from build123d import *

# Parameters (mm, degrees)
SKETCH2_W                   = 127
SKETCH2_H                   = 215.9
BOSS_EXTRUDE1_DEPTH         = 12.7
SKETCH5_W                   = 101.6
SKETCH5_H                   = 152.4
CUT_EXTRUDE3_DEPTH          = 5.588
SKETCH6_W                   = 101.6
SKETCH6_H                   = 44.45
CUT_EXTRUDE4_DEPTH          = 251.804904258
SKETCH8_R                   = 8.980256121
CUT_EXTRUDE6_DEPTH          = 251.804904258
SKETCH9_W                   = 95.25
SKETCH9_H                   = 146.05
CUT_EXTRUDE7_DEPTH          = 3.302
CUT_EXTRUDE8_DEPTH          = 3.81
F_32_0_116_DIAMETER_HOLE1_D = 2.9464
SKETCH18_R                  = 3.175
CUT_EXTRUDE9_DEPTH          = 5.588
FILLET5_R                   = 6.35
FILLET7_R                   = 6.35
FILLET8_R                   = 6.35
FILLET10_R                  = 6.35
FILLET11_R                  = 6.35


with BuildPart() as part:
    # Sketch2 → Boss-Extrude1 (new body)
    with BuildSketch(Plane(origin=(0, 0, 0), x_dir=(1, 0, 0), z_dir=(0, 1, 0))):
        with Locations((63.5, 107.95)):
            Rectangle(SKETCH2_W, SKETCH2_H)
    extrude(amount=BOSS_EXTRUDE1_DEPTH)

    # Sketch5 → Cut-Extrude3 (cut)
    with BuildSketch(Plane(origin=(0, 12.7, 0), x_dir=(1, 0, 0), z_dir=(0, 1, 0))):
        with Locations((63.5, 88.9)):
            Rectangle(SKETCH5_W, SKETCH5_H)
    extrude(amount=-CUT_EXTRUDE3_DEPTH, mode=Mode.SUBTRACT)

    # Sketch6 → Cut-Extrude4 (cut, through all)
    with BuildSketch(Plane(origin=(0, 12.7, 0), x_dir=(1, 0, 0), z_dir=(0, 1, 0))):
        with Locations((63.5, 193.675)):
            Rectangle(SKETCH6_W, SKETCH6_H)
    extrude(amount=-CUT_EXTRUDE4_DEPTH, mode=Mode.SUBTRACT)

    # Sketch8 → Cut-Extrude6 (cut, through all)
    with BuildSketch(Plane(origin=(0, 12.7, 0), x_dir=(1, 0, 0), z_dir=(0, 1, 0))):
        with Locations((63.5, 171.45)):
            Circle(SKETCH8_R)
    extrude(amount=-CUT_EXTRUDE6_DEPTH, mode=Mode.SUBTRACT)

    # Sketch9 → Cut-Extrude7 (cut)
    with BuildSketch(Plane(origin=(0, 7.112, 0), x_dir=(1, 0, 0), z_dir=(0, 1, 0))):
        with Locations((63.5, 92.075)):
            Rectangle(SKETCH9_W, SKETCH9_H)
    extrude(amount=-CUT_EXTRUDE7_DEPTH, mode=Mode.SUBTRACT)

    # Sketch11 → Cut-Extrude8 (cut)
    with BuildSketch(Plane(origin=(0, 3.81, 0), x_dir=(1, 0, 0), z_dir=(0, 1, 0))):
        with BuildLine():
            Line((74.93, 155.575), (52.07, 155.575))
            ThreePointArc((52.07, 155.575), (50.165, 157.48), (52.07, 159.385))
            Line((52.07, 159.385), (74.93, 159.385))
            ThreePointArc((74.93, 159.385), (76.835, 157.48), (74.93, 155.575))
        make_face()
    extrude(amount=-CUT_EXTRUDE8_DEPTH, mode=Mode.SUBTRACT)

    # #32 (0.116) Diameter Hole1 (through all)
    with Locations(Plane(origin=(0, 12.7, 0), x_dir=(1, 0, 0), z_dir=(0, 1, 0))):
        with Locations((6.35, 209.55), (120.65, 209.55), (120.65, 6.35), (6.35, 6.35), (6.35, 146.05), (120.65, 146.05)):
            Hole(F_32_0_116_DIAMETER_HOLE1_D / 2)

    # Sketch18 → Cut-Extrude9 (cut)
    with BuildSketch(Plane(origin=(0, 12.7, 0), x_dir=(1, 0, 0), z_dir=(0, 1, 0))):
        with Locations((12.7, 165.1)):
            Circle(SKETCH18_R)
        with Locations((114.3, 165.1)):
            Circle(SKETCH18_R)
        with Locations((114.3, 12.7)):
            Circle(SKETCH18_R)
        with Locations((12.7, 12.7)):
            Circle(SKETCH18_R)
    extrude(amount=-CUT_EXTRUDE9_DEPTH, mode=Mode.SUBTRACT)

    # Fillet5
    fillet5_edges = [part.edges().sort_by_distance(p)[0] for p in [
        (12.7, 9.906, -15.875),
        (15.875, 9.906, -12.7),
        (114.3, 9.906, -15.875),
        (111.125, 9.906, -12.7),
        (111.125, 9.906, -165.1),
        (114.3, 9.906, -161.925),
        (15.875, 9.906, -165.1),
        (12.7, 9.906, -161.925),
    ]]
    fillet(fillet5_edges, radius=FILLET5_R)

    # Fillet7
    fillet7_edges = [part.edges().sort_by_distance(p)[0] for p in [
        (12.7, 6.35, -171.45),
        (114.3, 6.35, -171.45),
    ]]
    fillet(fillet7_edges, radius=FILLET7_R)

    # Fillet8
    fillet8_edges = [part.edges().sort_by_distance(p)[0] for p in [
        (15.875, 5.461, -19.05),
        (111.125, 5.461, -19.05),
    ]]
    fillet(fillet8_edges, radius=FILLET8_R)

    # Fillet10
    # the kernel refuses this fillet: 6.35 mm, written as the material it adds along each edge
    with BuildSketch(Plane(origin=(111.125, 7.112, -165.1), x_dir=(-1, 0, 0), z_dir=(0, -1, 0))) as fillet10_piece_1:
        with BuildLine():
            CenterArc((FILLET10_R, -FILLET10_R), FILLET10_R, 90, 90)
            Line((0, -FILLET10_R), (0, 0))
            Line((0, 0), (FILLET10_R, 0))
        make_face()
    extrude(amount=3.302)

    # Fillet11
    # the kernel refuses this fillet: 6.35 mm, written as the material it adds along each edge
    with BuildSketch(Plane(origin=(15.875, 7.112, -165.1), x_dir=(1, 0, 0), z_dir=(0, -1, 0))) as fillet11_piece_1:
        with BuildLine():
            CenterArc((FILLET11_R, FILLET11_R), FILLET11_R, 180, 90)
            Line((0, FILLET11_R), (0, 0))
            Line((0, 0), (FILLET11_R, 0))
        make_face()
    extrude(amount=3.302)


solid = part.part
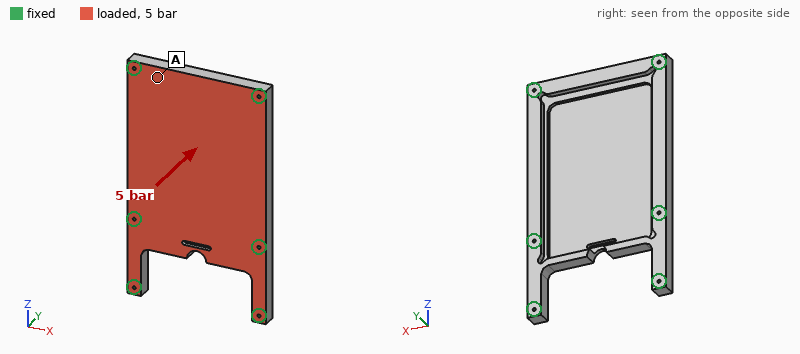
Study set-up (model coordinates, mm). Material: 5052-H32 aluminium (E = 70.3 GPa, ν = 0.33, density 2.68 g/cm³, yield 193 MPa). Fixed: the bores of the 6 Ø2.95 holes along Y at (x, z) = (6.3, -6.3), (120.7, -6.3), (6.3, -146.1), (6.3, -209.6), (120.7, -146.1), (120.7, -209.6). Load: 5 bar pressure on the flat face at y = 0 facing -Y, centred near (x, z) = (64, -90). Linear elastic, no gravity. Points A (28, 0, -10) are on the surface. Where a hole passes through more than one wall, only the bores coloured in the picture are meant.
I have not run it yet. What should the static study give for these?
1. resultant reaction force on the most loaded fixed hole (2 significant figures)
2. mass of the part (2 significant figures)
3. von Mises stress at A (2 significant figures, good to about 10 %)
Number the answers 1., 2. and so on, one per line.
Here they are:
1. 4.4 kN
2. 420 g
3. 21 MPa
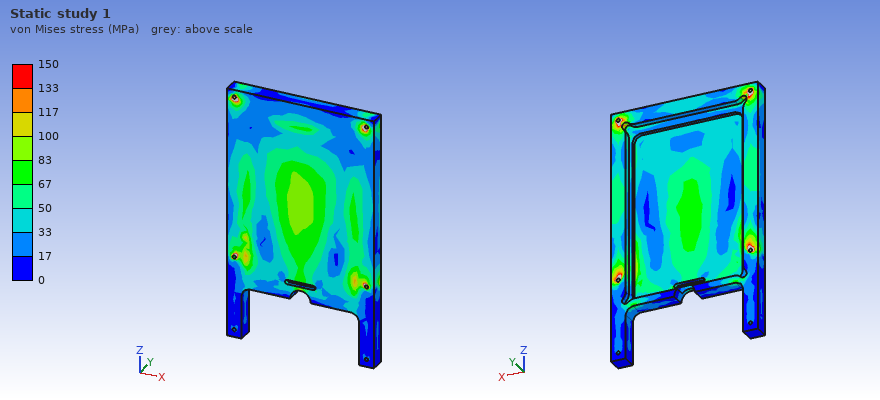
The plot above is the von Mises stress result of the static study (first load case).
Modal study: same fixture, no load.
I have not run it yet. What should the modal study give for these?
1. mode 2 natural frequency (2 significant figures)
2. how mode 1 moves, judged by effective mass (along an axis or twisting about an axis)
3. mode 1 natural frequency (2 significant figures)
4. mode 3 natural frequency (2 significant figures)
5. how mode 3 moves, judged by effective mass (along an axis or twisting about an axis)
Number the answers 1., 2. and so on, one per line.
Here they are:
1. 2700 Hz
2. along Y
3. 1800 Hz
4. 2800 Hz
5. twisting about Z
